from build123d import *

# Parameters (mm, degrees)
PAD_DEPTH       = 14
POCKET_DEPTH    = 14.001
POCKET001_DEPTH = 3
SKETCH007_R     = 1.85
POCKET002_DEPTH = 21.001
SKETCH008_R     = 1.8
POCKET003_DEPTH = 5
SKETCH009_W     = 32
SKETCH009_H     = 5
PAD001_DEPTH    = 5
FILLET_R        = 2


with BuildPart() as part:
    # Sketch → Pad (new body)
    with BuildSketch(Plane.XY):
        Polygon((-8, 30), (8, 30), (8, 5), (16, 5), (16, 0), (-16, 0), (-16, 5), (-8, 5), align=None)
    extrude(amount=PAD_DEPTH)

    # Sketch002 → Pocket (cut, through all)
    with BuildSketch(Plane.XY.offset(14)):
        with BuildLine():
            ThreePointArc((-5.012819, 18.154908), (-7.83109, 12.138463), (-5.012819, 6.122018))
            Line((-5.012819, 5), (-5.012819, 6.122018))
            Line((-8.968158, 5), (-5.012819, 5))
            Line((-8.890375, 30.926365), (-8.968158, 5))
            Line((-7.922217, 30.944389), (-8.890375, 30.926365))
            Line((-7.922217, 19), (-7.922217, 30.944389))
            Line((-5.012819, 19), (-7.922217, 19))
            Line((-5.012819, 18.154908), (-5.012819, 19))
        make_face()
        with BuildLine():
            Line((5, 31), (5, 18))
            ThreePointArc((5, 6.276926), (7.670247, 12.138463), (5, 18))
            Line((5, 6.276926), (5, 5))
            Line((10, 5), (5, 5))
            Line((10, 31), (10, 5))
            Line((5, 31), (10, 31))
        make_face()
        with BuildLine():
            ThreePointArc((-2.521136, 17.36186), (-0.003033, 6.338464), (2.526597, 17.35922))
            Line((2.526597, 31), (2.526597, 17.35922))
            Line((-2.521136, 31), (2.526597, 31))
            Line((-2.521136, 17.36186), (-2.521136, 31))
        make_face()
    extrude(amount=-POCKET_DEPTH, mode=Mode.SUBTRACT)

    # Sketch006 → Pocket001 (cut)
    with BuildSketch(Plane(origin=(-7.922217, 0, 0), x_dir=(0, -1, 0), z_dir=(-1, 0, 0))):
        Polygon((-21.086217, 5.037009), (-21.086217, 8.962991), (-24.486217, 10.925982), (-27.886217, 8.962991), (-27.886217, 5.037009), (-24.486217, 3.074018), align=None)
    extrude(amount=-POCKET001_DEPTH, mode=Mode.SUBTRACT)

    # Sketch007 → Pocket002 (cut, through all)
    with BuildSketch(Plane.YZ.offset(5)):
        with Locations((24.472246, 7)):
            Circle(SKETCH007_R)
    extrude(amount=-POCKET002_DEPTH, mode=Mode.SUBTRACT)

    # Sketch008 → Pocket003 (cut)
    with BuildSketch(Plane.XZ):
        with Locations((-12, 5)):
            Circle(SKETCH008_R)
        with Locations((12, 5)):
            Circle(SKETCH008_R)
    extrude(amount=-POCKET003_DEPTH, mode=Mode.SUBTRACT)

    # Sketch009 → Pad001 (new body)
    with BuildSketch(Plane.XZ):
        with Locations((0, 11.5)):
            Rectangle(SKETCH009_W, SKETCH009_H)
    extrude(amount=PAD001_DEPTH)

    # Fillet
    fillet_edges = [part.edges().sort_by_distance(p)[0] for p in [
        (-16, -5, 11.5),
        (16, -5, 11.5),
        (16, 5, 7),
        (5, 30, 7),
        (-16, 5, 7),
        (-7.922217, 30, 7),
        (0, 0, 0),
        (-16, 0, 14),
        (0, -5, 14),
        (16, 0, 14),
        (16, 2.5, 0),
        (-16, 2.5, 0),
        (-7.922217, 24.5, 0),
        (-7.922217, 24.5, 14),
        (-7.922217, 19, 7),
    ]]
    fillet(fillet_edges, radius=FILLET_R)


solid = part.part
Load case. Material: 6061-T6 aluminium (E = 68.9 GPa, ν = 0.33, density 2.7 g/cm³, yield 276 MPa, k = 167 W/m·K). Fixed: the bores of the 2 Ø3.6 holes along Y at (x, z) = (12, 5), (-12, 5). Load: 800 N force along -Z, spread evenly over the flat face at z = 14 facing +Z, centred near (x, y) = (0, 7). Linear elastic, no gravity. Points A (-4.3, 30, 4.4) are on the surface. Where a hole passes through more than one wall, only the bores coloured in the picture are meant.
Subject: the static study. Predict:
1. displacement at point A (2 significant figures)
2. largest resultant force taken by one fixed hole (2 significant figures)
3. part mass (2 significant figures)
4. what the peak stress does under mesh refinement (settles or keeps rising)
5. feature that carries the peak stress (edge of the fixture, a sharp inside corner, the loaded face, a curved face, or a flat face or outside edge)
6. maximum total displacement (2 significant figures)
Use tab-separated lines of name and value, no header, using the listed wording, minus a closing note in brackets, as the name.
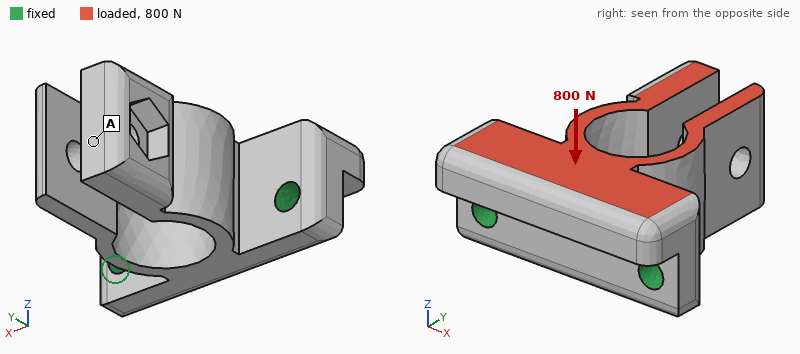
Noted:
displacement at point A	71 µm
largest resultant force taken by one fixed hole	440 N
part mass	13 g
what the peak stress does under mesh refinement	keeps rising
feature that carries the peak stress	a sharp inside corner
maximum total displacement	79 µm
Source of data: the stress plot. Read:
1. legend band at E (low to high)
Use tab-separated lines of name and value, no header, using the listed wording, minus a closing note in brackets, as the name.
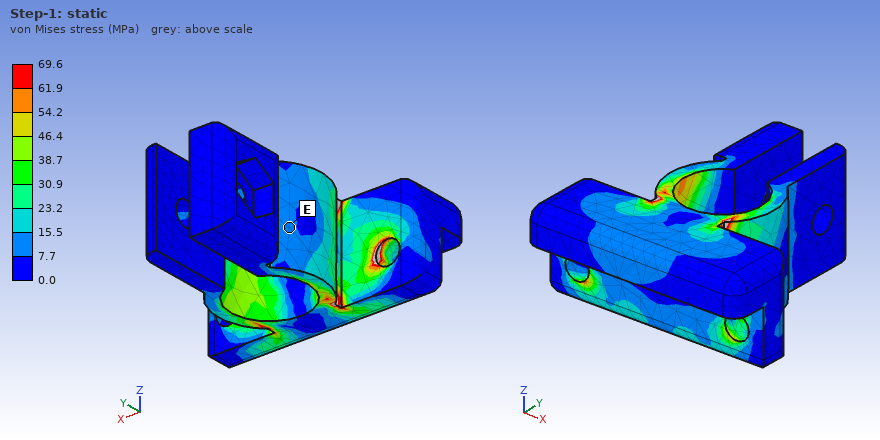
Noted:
legend band at E	7.7 to 15.5 MPa
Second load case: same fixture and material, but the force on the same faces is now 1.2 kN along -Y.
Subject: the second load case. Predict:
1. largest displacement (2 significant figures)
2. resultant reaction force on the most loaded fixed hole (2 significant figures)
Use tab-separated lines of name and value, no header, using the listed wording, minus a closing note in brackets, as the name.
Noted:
largest displacement	0.13 mm
resultant reaction force on the most loaded fixed hole	610 N
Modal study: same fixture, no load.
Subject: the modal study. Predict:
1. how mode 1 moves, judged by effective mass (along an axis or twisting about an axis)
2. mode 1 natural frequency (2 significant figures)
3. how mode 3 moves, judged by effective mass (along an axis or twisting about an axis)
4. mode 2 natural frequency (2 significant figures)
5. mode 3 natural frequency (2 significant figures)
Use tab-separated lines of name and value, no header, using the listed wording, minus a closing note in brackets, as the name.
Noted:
how mode 1 moves, judged by effective mass	along X
mode 1 natural frequency	1900 Hz
how mode 3 moves, judged by effective mass	along Z
mode 2 natural frequency	2400 Hz
mode 3 natural frequency	4900 Hz
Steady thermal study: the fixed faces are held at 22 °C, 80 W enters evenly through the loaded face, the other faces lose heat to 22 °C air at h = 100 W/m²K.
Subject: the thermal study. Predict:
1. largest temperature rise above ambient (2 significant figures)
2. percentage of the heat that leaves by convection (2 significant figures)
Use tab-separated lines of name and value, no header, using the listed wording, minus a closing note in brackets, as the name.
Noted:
largest temperature rise above ambient	57 K
percentage of the heat that leaves by convection	11 %
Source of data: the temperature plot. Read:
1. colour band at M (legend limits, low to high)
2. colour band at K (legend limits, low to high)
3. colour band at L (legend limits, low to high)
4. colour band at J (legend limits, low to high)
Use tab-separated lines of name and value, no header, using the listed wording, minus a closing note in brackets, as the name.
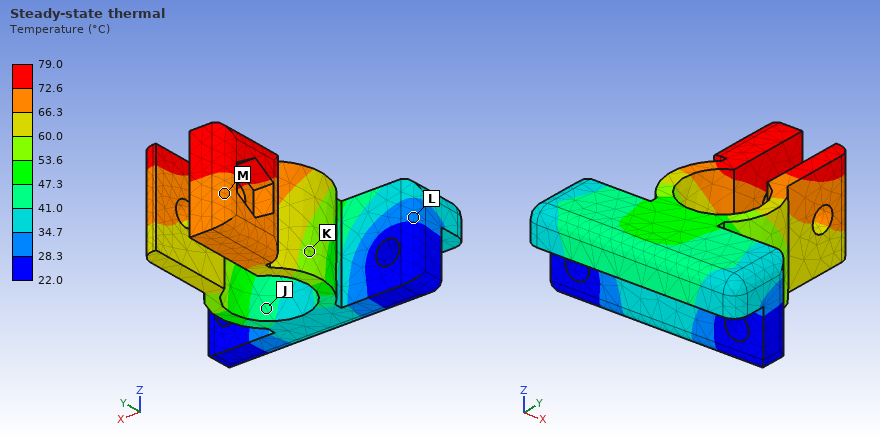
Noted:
colour band at M	66.3 to 72.6 °C
colour band at K	53.6 to 60.0 °C
colour band at L	28.3 to 34.7 °C
colour band at J	41.0 to 47.3 °C
